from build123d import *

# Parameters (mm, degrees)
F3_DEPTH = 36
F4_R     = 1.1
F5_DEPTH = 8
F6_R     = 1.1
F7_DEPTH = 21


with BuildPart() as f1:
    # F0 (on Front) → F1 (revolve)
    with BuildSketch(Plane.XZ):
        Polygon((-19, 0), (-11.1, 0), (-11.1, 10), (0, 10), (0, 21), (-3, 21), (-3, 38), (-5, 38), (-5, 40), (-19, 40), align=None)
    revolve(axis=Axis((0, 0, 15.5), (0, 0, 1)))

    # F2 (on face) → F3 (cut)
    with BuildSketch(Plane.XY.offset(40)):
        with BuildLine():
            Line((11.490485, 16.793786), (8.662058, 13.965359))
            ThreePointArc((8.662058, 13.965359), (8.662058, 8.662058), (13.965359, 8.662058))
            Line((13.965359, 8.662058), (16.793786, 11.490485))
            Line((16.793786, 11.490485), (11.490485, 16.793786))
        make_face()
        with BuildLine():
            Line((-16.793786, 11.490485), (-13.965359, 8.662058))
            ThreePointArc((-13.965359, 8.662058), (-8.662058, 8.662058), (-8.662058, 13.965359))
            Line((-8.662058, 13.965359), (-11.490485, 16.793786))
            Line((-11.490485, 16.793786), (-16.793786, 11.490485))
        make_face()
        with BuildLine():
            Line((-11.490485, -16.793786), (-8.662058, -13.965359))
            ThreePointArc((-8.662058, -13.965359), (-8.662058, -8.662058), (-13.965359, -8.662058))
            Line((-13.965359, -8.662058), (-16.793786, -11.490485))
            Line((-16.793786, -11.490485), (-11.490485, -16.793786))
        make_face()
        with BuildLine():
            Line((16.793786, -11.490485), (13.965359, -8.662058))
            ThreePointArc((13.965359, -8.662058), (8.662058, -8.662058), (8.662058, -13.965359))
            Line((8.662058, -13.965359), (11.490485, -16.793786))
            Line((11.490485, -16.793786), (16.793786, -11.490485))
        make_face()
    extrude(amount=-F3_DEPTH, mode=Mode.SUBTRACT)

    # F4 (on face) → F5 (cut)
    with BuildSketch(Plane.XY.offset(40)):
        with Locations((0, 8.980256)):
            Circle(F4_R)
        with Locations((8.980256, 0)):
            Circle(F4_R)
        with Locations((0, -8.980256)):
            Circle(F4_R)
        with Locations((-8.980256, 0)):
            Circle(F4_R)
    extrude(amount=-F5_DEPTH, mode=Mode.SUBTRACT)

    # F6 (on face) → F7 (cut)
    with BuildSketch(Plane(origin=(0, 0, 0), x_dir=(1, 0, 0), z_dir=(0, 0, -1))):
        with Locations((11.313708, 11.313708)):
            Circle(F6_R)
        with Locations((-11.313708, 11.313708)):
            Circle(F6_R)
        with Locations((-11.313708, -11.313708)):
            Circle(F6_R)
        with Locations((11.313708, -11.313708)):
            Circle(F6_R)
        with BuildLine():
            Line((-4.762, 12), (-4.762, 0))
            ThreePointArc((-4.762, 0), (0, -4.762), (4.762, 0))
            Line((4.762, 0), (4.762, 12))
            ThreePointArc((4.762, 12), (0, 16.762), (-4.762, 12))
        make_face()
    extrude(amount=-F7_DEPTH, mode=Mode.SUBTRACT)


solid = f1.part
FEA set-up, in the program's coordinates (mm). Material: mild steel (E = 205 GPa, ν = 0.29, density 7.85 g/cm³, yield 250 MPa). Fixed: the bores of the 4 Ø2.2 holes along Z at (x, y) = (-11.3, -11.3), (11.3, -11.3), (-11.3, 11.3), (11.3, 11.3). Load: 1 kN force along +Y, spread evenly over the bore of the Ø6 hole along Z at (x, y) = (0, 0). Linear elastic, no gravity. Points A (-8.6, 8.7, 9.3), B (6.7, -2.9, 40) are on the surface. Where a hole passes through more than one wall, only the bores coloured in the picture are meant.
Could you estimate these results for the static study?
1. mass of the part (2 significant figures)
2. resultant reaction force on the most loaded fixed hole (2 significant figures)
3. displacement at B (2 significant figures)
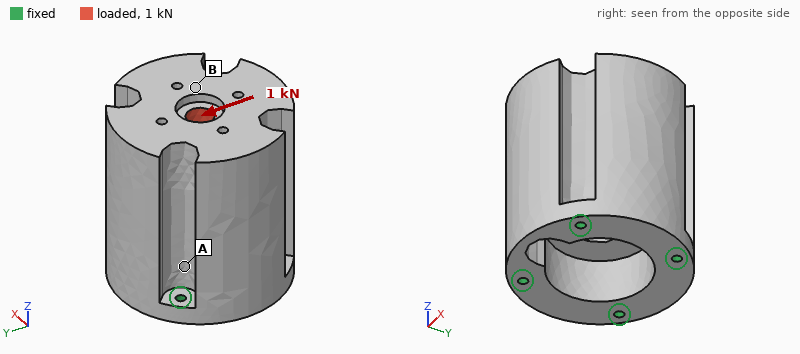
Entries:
250 g
650 N
5.6 µm
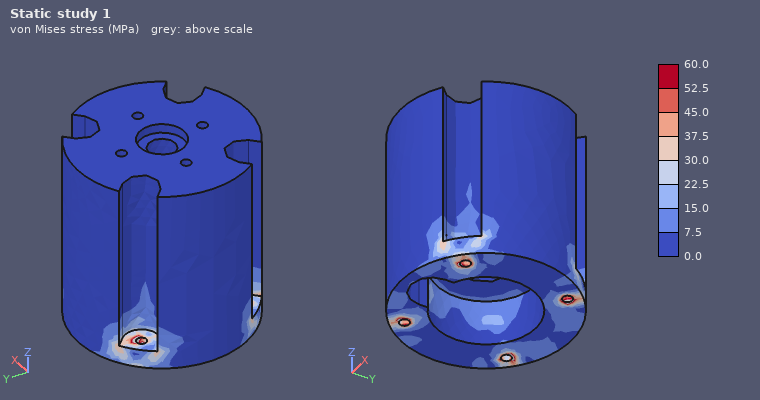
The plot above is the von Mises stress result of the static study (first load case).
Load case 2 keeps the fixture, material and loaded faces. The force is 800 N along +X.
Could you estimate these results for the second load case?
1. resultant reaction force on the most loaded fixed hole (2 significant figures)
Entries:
550 N
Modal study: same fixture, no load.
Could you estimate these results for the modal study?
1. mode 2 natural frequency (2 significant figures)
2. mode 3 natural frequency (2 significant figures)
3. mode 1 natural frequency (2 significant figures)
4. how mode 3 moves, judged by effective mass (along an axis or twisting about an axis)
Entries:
5700 Hz
14 kHz
5500 Hz
along Z
